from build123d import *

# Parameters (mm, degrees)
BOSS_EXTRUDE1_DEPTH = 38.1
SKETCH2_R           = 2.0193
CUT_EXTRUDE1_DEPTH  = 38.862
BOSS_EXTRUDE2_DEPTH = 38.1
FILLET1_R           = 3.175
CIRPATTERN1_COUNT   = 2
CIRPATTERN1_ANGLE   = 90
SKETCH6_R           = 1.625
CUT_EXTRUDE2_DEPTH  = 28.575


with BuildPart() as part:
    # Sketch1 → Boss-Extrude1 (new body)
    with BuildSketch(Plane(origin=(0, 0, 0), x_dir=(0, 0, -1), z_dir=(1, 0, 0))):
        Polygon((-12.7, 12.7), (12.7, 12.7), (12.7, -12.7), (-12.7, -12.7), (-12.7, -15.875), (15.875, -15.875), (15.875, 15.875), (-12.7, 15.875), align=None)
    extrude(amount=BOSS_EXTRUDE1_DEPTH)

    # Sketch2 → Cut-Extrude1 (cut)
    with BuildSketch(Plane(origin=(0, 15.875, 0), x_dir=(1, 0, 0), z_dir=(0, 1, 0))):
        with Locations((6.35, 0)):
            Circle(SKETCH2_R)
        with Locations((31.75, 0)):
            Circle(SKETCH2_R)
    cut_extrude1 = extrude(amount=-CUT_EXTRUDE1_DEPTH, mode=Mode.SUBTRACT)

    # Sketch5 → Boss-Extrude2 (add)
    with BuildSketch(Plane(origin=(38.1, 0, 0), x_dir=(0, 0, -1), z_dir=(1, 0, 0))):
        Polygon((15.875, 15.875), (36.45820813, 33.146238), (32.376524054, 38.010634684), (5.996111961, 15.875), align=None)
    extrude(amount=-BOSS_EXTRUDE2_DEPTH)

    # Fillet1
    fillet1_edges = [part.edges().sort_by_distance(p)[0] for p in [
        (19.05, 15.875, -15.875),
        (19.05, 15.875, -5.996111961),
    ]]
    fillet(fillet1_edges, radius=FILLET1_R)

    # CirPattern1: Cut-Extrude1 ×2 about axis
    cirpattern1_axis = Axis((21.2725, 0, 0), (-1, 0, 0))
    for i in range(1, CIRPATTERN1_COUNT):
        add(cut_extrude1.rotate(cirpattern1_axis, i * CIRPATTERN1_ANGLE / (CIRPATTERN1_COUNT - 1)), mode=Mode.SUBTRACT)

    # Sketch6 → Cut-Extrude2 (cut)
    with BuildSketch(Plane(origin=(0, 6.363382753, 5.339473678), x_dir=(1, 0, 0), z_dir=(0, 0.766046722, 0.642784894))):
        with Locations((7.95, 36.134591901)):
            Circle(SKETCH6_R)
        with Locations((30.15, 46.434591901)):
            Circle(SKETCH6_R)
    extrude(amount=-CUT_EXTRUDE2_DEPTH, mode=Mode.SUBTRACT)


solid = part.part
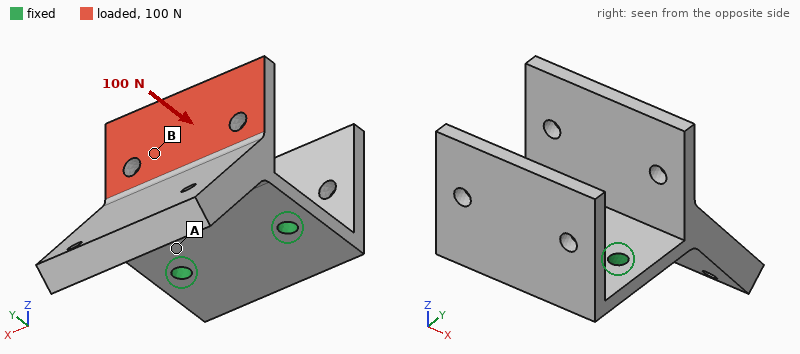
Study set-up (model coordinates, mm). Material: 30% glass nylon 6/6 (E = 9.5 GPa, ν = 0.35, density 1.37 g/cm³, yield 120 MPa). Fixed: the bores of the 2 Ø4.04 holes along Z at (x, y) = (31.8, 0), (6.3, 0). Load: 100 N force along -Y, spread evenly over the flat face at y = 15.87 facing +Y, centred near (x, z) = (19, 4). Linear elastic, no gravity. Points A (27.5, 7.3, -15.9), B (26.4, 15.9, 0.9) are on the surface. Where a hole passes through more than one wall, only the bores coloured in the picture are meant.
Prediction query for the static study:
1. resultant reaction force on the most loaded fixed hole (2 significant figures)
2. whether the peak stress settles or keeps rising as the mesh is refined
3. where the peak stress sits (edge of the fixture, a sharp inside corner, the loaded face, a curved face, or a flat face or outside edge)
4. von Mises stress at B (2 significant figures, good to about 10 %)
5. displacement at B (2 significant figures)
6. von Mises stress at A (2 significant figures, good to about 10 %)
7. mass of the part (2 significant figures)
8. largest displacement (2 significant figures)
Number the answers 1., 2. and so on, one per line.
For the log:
1. 51 N
2. keeps rising
3. edge of the fixture
4. 7.0 MPa
5. 0.48 mm
6. 25 MPa
7. 23 g
8. 0.89 mm
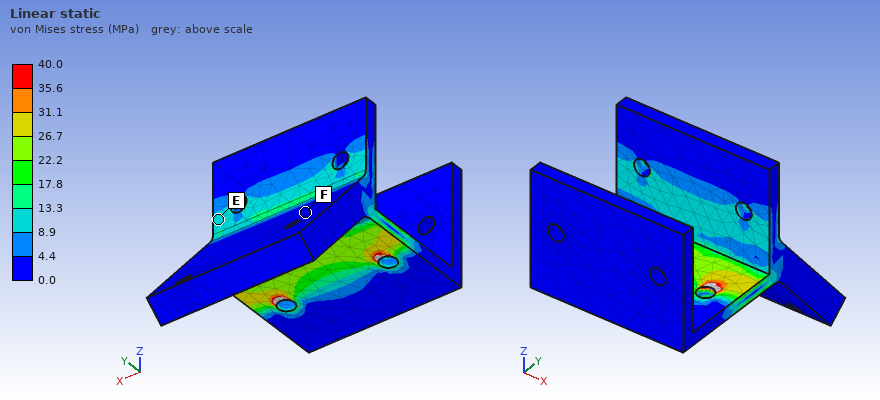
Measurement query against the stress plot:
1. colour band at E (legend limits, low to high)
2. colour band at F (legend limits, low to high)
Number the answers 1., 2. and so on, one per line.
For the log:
1. 8.9 to 13.3 MPa
2. 0.0 to 4.4 MPa
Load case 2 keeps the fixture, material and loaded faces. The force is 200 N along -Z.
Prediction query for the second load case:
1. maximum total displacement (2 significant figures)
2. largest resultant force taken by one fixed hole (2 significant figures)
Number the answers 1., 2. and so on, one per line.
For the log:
1. 0.90 mm
2. 100 N
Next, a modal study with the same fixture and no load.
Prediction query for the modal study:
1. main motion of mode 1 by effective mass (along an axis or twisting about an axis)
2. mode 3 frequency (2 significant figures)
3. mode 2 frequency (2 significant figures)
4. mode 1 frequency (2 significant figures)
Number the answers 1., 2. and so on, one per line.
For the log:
1. along Z
2. 1700 Hz
3. 1100 Hz
4. 530 Hz
